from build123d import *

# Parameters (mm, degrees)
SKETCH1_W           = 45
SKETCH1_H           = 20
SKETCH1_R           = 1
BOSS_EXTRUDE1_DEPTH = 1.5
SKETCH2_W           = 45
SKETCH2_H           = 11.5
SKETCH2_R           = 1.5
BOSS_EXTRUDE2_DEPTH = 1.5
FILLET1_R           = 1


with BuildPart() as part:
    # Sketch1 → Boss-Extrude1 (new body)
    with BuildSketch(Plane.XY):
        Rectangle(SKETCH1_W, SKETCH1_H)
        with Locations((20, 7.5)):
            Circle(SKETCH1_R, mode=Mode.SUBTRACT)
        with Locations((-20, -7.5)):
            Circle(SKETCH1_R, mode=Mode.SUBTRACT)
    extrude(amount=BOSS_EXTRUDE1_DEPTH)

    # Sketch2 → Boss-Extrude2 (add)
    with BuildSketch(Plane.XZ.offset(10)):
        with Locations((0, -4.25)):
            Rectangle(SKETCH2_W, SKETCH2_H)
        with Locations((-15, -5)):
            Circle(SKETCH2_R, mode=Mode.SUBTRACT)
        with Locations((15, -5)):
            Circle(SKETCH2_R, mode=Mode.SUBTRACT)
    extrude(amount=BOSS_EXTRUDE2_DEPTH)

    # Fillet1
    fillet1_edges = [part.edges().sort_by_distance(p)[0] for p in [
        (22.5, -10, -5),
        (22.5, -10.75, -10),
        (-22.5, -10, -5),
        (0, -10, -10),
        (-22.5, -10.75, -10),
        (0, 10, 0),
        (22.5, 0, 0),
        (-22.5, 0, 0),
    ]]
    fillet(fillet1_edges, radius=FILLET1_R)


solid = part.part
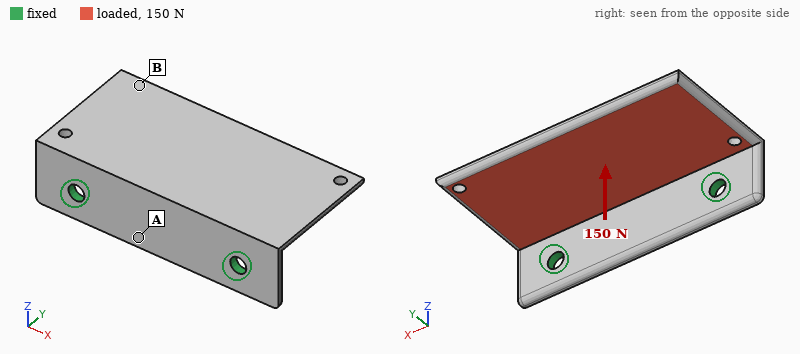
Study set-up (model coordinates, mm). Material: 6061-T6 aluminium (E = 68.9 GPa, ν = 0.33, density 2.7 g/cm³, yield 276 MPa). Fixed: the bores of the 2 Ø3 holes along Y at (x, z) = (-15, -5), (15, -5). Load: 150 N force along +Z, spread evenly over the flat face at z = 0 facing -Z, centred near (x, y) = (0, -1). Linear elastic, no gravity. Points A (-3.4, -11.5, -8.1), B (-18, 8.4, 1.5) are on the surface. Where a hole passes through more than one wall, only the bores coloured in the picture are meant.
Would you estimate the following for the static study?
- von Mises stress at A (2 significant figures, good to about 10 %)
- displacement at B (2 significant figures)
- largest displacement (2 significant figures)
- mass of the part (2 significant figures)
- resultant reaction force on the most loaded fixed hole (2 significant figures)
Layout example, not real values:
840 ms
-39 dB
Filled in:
36 MPa
0.36 mm
0.40 mm
5.6 g
76 N
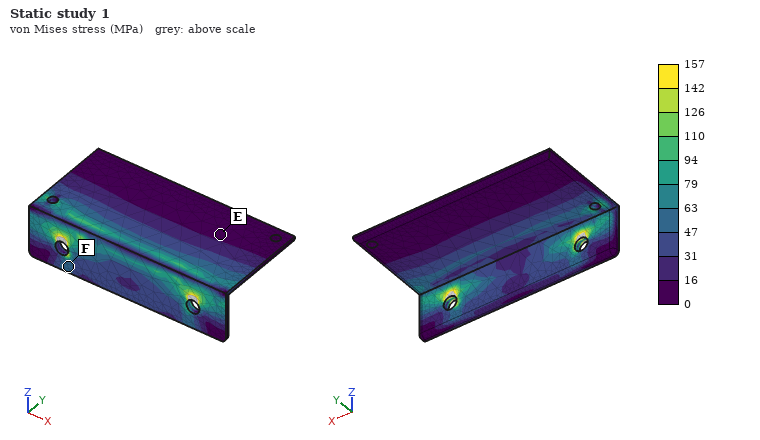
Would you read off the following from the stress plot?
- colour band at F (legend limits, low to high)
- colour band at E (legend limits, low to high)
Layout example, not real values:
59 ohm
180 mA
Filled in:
47 to 63 MPa
0 to 16 MPa
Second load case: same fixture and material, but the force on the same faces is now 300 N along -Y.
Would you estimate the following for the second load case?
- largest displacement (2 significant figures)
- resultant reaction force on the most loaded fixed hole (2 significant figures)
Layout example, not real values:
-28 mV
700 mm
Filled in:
75 µm
150 N
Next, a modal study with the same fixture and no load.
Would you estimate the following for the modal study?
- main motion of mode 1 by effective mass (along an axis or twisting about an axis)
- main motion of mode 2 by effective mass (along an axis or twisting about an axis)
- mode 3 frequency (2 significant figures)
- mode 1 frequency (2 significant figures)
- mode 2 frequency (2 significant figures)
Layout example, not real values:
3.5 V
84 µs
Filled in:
along Z
twisting about Y
7100 Hz
2000 Hz
3500 Hz
